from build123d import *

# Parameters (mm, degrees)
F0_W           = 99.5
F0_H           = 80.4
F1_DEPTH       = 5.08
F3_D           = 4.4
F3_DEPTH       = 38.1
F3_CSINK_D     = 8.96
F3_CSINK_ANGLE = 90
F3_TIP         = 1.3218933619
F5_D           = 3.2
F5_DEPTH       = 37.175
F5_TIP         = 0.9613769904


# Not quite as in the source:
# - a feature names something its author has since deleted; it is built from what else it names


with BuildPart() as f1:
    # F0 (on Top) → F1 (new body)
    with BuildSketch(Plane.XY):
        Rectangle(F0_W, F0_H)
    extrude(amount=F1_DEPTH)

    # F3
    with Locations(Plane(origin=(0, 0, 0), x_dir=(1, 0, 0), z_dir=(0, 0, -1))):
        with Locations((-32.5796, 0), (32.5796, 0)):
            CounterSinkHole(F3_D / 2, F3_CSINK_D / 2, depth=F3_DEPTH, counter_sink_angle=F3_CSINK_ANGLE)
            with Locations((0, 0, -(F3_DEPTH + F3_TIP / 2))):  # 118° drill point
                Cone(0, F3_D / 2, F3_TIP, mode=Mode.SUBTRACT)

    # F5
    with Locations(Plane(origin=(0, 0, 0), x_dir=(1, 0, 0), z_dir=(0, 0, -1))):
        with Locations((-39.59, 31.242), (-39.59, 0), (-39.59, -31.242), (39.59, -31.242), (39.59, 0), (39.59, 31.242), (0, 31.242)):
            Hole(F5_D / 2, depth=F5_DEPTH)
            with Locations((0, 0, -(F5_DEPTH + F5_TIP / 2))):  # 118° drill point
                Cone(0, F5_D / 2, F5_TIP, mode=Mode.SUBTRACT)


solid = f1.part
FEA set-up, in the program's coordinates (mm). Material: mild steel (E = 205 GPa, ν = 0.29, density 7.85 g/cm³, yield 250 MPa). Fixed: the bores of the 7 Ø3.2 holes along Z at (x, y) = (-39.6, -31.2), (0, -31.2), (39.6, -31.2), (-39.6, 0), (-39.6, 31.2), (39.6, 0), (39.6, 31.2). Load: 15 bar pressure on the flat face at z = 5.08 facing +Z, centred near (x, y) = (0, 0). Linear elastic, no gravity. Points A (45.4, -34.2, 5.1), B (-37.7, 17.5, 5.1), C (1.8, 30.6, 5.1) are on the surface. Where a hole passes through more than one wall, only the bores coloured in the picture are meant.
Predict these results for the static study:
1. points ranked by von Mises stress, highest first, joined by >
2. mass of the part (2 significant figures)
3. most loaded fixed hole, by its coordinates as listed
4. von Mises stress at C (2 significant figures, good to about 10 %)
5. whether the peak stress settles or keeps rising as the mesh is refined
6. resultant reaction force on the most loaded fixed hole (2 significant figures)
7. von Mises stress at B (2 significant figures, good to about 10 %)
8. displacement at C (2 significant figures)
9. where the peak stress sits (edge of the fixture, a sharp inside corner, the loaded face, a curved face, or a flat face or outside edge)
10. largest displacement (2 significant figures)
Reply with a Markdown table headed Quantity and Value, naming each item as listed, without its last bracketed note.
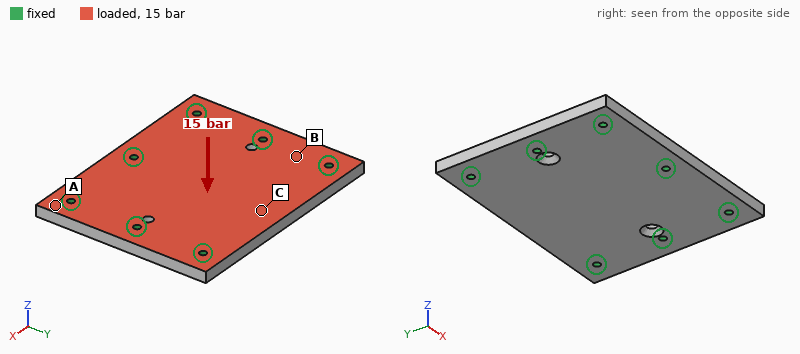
| Quantity | Value |
|---|---|
| points ranked by von Mises stress, highest first, joined by > | C > B > A |
| mass of the part | 310 g |
| most loaded fixed hole, by its coordinates as listed | (0, -31.2) |
| von Mises stress at C | 90 MPa |
| whether the peak stress settles or keeps rising as the mesh is refined | keeps rising |
| resultant reaction force on the most loaded fixed hole | 2.4 kN |
| von Mises stress at B | 58 MPa |
| displacement at C | 82 µm |
| where the peak stress sits | edge of the fixture |
| largest displacement | 90 µm |
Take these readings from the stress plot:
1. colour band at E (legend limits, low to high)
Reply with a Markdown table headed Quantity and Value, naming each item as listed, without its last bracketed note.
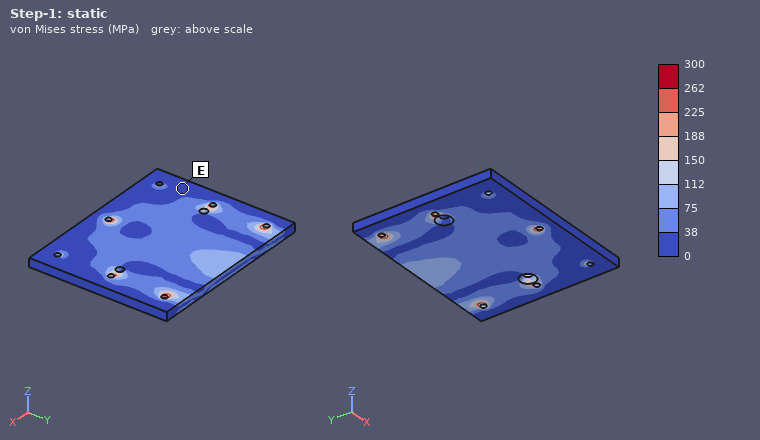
| Quantity | Value |
|---|---|
| colour band at E | 0 to 38 MPa |
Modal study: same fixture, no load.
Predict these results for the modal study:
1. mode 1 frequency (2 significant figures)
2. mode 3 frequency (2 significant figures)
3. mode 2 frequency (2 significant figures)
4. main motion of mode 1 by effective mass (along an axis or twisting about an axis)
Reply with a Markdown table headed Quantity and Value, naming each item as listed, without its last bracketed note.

| Quantity | Value |
|---|---|
| mode 1 frequency | 4100 Hz |
| mode 3 frequency | 10 kHz |
| mode 2 frequency | 7400 Hz |
| main motion of mode 1 by effective mass | along Z |
